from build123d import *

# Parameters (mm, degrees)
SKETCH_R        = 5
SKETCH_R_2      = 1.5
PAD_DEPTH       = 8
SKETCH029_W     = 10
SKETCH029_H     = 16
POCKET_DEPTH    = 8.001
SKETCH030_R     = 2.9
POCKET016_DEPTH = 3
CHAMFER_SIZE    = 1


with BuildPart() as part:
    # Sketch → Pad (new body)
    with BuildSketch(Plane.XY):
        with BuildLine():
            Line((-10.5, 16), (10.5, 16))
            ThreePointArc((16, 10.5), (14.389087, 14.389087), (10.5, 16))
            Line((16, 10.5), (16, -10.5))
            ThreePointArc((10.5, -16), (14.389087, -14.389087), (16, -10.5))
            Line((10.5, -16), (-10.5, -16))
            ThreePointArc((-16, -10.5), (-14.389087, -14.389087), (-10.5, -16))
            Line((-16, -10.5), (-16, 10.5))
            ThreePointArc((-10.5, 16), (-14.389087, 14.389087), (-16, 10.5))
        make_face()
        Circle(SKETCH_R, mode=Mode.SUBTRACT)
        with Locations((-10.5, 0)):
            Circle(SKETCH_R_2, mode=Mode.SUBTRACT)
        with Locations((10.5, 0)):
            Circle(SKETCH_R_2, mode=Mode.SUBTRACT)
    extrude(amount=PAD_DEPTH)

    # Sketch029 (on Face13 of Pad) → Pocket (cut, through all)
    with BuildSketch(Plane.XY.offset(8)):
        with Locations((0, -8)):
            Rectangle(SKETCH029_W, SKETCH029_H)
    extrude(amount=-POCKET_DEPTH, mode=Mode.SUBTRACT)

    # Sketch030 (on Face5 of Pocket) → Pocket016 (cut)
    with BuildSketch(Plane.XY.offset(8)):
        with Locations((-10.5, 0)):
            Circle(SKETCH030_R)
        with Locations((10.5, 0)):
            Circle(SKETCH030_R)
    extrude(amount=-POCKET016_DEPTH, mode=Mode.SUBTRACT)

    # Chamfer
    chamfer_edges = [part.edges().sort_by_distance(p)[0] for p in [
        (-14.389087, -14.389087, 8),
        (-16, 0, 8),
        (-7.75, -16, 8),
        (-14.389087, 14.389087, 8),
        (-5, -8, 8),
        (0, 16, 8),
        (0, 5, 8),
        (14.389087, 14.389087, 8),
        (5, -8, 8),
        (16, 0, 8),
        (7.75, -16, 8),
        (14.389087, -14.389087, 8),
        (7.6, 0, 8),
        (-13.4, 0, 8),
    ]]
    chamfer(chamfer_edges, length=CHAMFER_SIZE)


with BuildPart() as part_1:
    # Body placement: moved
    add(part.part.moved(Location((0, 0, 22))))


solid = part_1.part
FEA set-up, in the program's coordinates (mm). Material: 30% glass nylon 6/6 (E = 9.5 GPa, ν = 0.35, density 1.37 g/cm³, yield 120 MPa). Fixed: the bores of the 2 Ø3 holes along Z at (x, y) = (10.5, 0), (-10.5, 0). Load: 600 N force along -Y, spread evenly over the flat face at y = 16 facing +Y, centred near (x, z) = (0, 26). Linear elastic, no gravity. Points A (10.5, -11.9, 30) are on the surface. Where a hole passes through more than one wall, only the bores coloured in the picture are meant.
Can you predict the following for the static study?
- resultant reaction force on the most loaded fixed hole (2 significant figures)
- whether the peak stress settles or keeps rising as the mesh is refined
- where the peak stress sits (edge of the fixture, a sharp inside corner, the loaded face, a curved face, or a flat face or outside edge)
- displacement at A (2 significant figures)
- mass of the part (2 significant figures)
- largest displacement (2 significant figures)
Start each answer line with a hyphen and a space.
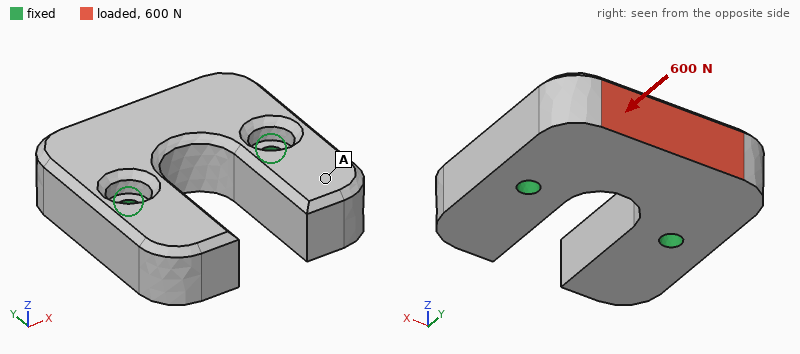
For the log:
- 320 N
- keeps rising
- edge of the fixture
- 7.1 µm
- 8.3 g
- 13 µm
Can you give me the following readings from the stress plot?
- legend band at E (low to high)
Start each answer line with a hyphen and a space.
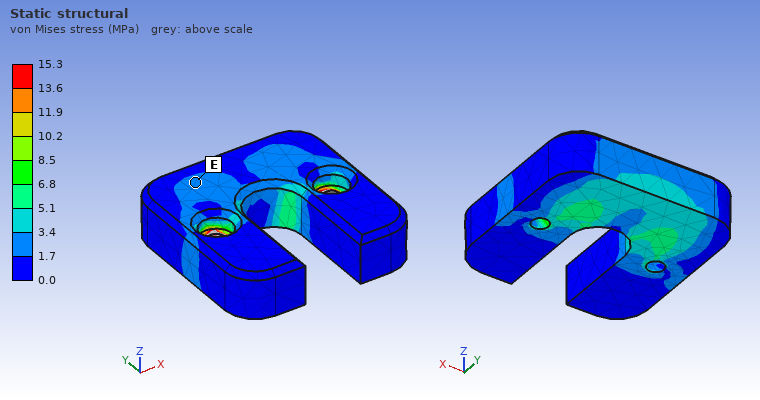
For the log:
- 1.7 to 3.4 MPa
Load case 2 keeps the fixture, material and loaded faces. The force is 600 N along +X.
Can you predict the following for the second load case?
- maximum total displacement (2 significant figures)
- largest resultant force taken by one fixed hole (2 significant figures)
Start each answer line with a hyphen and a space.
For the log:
- 29 µm
- 500 N
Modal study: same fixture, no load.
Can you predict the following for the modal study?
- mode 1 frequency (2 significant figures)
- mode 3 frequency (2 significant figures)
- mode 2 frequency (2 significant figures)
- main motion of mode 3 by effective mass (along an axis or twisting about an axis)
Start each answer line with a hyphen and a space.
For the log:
- 6000 Hz
- 10000 Hz
- 8400 Hz
- along Z
